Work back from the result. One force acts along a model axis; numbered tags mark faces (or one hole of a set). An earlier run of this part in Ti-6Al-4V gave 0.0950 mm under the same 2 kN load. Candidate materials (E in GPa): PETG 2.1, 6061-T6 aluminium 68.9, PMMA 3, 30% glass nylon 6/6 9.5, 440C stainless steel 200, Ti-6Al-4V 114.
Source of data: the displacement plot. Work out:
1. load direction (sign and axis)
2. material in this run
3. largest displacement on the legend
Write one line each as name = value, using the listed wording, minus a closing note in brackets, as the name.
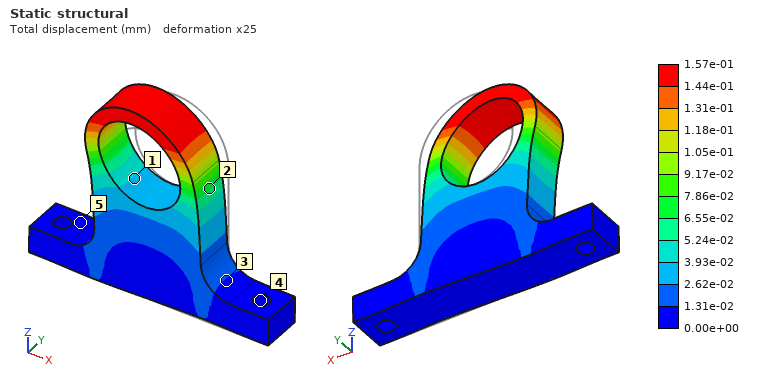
load direction = -X
material in this run = 6061-T6 aluminium
largest displacement on the legend = 1.57e-01 mm
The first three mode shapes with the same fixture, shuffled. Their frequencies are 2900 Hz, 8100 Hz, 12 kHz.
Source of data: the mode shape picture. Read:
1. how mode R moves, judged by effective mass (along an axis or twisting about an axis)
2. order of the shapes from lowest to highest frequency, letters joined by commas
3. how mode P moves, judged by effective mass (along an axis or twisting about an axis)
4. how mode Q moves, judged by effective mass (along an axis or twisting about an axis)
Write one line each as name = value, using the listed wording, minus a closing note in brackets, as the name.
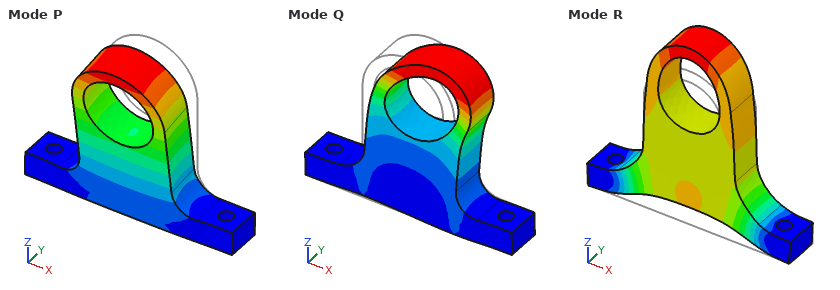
how mode R moves, judged by effective mass = along Z
order of the shapes from lowest to highest frequency, letters joined by commas = P, Q, R
how mode P moves, judged by effective mass = along Y
how mode Q moves, judged by effective mass = along X
